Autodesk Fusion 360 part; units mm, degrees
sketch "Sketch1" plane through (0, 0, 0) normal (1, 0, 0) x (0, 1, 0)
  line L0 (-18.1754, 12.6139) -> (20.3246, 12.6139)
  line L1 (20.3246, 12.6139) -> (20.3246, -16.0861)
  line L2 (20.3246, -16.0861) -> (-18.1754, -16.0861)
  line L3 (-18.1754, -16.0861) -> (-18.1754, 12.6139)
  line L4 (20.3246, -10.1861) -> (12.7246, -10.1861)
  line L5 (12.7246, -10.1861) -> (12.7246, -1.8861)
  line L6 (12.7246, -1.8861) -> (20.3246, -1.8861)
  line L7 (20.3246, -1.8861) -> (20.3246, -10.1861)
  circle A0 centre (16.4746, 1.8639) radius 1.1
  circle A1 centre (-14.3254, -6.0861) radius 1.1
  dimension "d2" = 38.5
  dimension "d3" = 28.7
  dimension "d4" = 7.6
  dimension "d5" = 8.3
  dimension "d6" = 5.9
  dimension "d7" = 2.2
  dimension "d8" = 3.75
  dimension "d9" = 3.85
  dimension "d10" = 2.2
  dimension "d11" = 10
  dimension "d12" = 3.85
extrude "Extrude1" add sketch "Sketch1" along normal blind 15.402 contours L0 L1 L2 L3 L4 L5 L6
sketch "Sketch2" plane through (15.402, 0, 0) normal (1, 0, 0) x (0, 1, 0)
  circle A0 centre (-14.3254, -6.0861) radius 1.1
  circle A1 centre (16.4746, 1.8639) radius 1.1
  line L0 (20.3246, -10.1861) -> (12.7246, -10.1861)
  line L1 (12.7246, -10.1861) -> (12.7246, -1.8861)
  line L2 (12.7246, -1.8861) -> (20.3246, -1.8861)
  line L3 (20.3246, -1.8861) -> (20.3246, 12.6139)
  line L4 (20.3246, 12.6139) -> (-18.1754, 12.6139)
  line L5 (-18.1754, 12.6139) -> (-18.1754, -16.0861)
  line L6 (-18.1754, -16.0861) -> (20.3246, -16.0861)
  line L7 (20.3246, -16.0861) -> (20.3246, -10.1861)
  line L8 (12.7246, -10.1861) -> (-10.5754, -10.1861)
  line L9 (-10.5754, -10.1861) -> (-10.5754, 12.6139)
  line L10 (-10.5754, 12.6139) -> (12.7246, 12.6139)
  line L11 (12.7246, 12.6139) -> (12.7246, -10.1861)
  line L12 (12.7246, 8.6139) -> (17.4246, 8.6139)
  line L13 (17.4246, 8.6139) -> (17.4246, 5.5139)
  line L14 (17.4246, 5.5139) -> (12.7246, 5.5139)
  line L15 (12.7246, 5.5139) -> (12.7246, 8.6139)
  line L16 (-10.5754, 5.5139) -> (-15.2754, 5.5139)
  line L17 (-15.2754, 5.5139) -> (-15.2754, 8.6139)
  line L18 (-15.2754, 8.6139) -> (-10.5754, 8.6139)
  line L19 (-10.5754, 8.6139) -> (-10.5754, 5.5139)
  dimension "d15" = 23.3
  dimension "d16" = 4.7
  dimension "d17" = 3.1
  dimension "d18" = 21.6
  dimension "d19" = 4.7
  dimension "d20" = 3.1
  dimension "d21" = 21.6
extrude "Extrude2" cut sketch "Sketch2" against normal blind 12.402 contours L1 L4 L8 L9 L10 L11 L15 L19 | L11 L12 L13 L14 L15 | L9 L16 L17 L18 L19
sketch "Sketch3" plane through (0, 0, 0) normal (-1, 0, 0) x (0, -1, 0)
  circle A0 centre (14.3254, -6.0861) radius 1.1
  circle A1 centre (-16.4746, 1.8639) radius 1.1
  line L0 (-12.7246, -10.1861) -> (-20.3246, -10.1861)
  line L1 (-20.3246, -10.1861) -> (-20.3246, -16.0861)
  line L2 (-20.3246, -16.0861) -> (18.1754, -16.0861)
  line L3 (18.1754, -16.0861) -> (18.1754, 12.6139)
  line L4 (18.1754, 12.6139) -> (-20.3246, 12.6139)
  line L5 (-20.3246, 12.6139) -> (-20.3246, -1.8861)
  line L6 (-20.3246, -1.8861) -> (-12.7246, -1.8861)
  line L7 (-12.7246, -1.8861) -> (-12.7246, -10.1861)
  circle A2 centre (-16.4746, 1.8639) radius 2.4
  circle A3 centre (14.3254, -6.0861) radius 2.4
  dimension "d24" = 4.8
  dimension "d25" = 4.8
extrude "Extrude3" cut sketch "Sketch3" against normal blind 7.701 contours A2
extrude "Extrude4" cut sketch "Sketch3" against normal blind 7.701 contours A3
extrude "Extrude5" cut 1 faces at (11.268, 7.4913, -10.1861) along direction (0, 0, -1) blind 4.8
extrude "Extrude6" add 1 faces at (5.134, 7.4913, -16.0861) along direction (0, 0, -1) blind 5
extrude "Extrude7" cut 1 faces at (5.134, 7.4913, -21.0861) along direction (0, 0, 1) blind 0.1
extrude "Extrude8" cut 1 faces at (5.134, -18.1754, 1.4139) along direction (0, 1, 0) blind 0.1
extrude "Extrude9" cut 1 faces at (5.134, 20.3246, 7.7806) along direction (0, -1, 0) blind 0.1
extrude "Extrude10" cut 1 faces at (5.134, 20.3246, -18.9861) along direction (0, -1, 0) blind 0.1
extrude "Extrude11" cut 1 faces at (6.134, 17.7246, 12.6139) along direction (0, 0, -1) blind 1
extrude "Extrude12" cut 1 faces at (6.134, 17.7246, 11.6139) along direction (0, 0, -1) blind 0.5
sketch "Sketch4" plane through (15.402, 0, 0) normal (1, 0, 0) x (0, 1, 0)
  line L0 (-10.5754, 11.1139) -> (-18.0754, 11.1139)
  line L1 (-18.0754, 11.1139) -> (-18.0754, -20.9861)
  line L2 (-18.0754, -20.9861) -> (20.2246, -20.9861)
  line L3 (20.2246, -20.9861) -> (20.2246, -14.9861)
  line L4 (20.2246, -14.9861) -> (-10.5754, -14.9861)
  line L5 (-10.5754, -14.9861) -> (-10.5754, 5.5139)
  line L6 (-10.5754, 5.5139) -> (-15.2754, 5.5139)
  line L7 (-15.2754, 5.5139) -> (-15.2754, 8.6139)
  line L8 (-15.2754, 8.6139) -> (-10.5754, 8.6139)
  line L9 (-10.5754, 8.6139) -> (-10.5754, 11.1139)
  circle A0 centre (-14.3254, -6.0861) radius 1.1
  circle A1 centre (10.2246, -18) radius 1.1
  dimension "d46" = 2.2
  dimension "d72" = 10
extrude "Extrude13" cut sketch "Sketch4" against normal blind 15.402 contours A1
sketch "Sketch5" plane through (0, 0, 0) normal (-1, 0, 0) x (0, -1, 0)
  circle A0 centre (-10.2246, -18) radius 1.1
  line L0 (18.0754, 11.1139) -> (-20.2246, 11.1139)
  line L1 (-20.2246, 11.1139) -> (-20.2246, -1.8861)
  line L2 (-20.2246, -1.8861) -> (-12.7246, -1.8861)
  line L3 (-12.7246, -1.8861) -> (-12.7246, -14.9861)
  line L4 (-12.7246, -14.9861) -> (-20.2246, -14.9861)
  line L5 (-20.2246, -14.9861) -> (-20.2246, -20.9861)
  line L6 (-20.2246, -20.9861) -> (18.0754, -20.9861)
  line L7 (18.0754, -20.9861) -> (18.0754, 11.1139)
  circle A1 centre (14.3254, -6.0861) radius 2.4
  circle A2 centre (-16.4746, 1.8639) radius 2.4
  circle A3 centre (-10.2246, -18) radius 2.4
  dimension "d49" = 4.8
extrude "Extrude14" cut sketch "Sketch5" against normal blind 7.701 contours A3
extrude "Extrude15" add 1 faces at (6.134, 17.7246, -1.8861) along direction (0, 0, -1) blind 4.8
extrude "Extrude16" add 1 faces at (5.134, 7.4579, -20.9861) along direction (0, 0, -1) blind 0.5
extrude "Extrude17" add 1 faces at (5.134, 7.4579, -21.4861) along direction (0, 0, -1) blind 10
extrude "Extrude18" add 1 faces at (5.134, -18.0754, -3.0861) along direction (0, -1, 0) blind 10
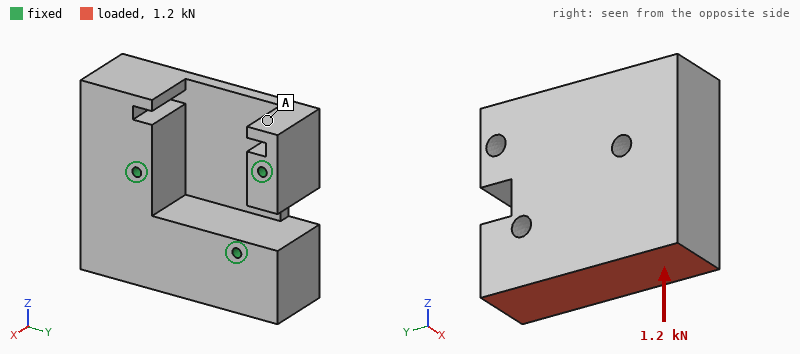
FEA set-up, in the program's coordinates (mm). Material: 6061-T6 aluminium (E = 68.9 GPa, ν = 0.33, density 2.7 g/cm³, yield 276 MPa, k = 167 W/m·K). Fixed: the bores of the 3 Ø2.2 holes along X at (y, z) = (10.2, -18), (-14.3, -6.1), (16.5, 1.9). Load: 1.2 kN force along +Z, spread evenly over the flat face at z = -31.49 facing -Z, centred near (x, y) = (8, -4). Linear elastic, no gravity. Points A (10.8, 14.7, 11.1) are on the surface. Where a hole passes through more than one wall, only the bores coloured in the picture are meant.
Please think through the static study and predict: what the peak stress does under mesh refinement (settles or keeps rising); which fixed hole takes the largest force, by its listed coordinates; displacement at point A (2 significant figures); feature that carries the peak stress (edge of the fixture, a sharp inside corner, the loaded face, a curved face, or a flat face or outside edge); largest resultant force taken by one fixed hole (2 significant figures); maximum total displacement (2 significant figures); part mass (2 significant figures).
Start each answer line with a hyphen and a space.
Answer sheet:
- keeps rising
- (-14.3, -6.1)
- 1.1 µm
- edge of the fixture
- 640 N
- 6.6 µm
- 60 g
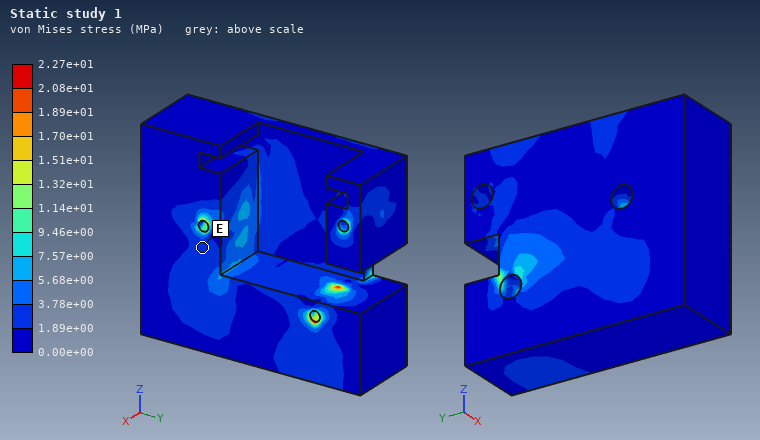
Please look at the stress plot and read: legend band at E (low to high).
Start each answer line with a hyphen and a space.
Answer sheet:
- 1.89e+00 to 3.78e+00 MPa
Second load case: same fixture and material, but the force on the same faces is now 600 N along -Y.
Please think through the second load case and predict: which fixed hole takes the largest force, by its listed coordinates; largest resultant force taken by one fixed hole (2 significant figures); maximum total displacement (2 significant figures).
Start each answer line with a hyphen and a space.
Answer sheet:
- (10.2, -18)
- 600 N
- 3.8 µm
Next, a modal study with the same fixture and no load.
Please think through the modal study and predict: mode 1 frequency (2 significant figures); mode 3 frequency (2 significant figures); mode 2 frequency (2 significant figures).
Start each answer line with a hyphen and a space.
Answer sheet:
- 7100 Hz
- 14 kHz
- 13 kHz
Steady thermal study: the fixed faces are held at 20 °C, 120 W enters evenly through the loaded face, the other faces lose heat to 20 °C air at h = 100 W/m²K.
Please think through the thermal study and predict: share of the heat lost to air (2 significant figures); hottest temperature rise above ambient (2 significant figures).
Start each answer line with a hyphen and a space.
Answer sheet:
- 7.6 %
- 33 K
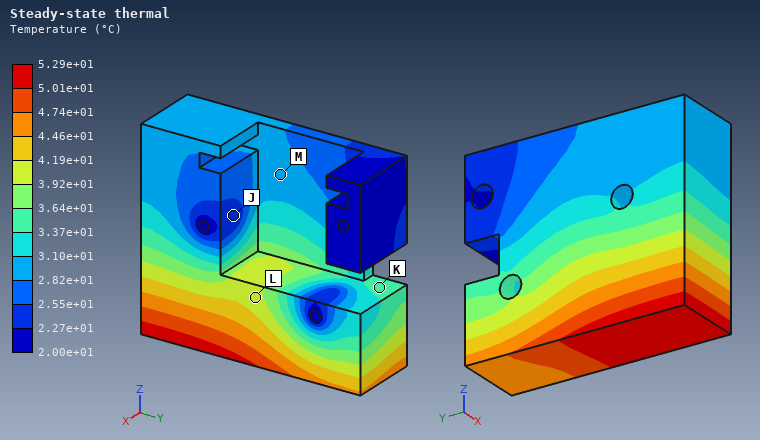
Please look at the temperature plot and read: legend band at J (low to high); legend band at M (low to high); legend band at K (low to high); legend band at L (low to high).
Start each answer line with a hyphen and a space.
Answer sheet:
- 2.27e+01 to 2.55e+01 °C
- 2.82e+01 to 3.10e+01 °C
- 3.37e+01 to 3.64e+01 °C
- 3.92e+01 to 4.19e+01 °C
